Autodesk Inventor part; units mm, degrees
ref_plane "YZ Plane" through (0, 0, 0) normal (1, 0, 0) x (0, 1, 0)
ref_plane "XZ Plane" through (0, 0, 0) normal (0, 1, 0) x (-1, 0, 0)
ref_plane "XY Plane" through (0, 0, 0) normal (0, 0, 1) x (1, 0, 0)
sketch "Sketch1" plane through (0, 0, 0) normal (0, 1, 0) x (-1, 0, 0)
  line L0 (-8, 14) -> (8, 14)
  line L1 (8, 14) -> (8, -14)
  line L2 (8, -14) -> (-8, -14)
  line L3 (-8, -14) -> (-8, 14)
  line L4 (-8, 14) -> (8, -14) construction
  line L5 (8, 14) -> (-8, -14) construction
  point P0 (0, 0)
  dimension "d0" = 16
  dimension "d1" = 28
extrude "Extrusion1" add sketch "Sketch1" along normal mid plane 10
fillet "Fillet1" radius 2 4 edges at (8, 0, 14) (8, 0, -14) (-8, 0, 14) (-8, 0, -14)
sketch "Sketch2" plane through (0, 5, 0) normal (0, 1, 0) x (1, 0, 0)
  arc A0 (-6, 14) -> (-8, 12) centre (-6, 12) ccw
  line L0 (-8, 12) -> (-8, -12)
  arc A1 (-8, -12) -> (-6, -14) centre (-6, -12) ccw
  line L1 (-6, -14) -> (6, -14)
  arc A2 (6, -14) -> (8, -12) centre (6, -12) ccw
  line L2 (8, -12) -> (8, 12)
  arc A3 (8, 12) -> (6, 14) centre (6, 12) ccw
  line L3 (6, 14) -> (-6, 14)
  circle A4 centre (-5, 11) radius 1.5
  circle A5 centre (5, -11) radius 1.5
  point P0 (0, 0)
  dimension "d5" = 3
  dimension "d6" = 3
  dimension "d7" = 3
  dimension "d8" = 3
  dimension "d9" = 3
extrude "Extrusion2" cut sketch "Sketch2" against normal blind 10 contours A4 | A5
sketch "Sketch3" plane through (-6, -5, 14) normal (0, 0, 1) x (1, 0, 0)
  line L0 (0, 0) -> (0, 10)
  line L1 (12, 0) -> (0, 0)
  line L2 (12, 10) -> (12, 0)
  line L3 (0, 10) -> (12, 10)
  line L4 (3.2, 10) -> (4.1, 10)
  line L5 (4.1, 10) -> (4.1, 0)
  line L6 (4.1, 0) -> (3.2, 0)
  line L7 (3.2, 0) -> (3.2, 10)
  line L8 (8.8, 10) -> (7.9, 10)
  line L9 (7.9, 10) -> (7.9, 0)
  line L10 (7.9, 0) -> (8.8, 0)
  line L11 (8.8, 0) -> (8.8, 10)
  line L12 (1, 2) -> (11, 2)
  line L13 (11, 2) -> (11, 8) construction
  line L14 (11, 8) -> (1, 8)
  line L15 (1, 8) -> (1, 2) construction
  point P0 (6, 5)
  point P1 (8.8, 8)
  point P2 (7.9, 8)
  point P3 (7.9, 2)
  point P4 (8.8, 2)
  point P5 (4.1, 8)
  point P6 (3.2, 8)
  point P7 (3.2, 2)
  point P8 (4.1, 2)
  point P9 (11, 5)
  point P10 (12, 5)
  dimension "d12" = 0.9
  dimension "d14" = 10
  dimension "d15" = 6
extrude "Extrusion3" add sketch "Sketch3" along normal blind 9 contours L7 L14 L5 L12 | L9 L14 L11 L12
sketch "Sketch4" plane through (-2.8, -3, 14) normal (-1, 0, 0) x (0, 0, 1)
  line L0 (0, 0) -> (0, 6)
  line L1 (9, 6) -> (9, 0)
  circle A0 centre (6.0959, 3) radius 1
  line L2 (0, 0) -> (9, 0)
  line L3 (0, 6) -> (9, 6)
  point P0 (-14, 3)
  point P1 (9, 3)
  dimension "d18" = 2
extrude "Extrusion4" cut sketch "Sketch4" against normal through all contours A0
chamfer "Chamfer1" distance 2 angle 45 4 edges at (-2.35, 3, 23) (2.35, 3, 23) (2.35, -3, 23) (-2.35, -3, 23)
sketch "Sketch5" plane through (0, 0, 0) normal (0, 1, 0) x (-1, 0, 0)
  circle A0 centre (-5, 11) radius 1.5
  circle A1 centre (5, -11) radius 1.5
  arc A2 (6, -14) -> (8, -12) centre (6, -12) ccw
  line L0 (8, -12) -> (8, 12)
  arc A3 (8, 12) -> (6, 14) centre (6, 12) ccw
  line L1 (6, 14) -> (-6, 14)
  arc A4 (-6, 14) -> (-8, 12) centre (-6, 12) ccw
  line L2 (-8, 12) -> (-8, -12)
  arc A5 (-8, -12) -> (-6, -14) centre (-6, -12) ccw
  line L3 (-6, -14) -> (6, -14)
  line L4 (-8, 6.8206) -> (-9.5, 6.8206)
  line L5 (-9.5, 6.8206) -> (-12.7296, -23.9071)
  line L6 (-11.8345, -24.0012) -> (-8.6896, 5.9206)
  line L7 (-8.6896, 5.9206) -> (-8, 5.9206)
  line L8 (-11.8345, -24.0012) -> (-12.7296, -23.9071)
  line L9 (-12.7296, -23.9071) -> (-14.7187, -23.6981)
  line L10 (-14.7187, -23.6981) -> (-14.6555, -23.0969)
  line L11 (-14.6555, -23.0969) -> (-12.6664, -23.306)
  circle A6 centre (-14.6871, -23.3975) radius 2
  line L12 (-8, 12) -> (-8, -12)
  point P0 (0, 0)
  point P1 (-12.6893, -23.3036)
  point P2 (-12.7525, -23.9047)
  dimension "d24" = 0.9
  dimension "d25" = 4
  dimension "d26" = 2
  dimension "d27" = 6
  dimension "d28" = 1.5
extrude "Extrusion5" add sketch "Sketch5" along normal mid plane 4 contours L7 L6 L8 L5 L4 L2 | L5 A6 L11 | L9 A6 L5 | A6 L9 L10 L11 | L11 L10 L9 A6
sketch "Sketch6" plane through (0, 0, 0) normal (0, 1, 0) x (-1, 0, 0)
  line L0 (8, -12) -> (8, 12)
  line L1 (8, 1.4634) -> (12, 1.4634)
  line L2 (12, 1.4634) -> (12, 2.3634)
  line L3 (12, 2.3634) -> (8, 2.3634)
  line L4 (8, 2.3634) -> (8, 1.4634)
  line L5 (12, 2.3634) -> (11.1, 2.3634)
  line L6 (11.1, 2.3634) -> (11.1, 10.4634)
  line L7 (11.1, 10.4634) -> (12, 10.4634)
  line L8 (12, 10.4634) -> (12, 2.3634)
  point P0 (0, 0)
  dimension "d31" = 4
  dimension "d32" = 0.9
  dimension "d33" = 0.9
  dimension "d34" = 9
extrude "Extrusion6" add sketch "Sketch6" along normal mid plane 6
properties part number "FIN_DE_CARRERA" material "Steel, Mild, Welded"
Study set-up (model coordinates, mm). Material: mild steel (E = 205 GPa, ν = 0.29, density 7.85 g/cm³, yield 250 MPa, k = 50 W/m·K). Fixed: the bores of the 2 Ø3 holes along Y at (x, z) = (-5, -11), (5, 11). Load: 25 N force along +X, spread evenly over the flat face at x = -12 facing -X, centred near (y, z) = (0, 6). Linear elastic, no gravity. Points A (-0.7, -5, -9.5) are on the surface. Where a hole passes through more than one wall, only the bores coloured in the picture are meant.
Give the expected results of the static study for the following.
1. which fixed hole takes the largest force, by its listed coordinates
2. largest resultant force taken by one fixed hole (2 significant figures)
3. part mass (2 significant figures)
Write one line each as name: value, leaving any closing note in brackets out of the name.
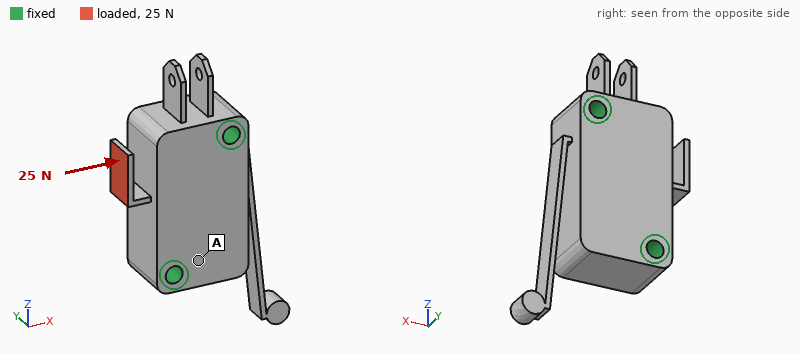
which fixed hole takes the largest force, by its listed coordinates: (5, 11)
largest resultant force taken by one fixed hole: 20 N
part mass: 36 g
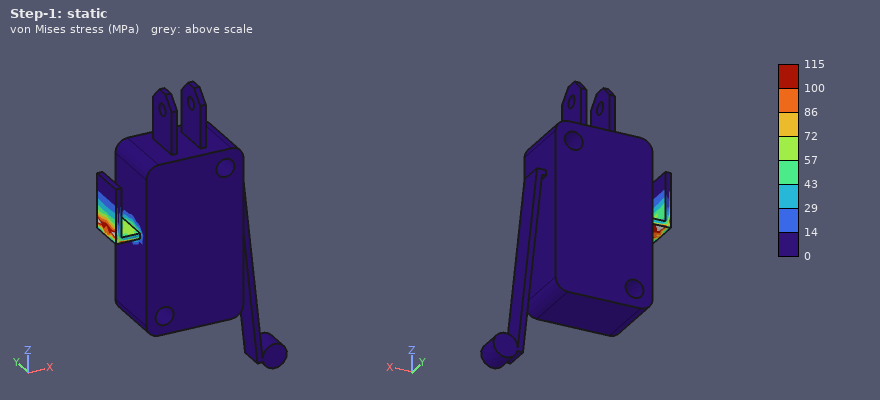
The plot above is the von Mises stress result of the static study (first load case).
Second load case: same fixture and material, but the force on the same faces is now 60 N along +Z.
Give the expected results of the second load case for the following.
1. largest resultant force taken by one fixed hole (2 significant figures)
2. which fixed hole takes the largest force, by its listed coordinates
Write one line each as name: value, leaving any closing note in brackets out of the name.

largest resultant force taken by one fixed hole: 48 N
which fixed hole takes the largest force, by its listed coordinates: (-5, -11)
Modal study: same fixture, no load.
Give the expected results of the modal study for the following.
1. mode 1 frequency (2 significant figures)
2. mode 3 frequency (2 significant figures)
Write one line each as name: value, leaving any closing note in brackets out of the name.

mode 1 frequency: 450 Hz
mode 3 frequency: 3400 Hz
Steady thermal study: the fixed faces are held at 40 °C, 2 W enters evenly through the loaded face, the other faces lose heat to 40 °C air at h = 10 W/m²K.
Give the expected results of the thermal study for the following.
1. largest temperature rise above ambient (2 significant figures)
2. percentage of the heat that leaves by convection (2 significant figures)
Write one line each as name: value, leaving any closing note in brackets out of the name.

largest temperature rise above ambient: 59 K
percentage of the heat that leaves by convection: 3.2 %
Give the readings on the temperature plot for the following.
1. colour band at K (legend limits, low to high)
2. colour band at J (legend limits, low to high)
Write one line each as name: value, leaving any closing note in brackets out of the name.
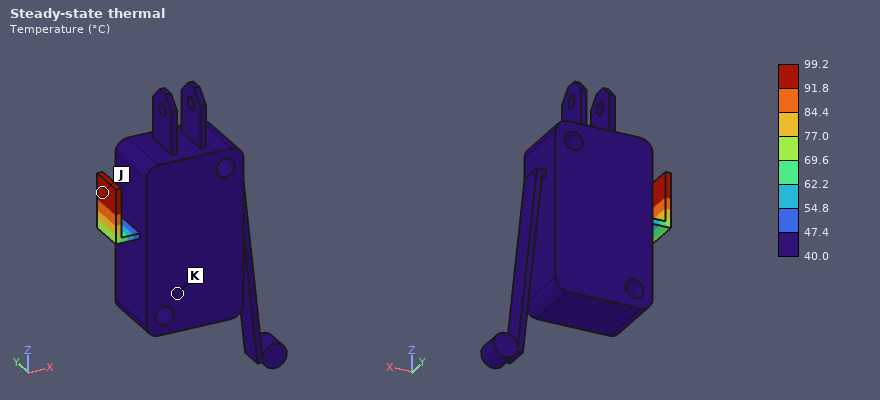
colour band at K: 40.0 to 47.4 °C
colour band at J: 91.8 to 99.2 °C
